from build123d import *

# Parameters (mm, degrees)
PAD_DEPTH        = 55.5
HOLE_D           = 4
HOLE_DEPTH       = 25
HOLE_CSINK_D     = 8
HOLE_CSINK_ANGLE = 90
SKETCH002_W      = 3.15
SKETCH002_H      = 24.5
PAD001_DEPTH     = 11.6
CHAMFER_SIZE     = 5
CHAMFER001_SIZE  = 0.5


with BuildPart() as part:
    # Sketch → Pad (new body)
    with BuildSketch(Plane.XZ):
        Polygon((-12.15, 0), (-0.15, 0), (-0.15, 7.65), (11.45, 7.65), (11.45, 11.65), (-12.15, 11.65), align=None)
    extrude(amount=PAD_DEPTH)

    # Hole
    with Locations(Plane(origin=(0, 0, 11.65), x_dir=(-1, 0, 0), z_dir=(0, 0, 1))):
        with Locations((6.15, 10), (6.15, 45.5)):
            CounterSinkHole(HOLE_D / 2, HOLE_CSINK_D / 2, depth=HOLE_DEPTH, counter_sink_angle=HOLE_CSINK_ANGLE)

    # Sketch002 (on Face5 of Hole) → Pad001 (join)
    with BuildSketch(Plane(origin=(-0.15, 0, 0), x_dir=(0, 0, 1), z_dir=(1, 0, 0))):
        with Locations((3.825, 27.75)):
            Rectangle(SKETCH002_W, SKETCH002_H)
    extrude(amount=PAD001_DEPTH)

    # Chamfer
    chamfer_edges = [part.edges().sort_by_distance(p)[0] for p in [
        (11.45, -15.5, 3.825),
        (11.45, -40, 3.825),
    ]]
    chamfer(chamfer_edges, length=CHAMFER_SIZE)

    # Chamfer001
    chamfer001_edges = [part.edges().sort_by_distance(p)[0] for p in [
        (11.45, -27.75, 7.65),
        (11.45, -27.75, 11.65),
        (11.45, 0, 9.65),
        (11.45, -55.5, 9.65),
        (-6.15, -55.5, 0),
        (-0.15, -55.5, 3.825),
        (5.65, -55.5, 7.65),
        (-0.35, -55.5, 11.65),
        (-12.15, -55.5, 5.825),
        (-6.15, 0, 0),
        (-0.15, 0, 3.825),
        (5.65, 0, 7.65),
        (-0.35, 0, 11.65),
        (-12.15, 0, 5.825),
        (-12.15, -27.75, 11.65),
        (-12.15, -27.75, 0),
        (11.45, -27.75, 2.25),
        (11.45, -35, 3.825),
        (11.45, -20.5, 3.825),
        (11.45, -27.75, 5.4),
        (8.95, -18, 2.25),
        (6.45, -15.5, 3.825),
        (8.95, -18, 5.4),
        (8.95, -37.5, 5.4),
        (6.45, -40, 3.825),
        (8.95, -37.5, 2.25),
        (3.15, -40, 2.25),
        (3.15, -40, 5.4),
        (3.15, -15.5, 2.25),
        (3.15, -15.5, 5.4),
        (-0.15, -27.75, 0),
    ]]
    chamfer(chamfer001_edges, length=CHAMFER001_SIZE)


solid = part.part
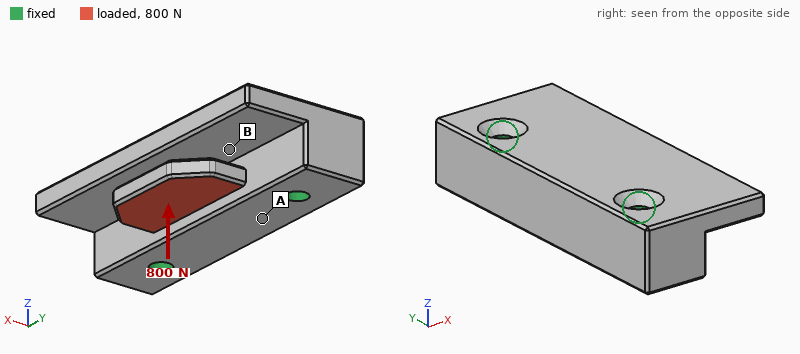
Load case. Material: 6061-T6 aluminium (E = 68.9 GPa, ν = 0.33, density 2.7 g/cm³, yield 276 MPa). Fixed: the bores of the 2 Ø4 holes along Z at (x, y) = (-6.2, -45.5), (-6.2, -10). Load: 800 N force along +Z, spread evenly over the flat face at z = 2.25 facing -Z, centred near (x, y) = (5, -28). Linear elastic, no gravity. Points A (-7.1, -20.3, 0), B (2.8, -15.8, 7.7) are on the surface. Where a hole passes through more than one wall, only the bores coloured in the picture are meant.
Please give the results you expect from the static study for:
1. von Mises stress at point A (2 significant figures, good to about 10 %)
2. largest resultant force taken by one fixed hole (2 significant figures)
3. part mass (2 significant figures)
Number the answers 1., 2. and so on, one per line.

1. 14 MPa
2. 400 N
3. 29 g
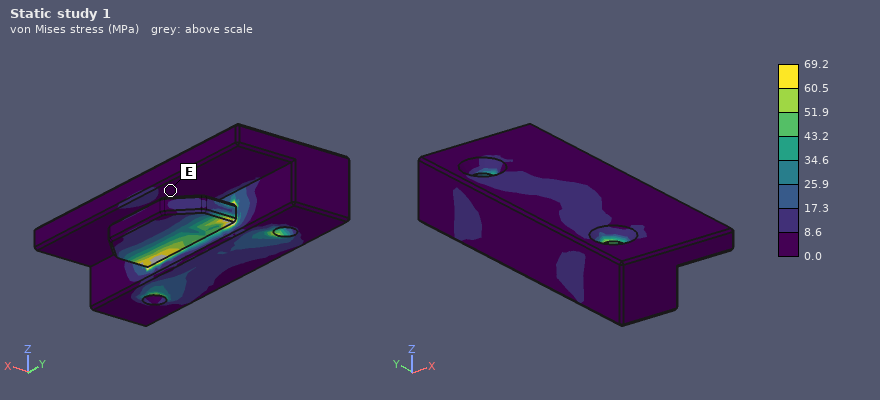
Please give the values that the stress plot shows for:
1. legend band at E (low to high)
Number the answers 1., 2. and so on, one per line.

1. 0.0 to 8.6 MPa
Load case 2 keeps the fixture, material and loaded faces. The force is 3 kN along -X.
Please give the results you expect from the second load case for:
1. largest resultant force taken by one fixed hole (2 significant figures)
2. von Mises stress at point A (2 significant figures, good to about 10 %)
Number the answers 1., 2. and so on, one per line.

1. 1.6 kN
2. 26 MPa
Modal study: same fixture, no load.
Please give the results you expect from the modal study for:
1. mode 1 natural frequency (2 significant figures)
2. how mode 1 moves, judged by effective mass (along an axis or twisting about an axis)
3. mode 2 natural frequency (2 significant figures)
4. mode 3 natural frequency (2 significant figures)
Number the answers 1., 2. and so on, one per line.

1. 13 kHz
2. along Z
3. 17 kHz
4. 17 kHz
